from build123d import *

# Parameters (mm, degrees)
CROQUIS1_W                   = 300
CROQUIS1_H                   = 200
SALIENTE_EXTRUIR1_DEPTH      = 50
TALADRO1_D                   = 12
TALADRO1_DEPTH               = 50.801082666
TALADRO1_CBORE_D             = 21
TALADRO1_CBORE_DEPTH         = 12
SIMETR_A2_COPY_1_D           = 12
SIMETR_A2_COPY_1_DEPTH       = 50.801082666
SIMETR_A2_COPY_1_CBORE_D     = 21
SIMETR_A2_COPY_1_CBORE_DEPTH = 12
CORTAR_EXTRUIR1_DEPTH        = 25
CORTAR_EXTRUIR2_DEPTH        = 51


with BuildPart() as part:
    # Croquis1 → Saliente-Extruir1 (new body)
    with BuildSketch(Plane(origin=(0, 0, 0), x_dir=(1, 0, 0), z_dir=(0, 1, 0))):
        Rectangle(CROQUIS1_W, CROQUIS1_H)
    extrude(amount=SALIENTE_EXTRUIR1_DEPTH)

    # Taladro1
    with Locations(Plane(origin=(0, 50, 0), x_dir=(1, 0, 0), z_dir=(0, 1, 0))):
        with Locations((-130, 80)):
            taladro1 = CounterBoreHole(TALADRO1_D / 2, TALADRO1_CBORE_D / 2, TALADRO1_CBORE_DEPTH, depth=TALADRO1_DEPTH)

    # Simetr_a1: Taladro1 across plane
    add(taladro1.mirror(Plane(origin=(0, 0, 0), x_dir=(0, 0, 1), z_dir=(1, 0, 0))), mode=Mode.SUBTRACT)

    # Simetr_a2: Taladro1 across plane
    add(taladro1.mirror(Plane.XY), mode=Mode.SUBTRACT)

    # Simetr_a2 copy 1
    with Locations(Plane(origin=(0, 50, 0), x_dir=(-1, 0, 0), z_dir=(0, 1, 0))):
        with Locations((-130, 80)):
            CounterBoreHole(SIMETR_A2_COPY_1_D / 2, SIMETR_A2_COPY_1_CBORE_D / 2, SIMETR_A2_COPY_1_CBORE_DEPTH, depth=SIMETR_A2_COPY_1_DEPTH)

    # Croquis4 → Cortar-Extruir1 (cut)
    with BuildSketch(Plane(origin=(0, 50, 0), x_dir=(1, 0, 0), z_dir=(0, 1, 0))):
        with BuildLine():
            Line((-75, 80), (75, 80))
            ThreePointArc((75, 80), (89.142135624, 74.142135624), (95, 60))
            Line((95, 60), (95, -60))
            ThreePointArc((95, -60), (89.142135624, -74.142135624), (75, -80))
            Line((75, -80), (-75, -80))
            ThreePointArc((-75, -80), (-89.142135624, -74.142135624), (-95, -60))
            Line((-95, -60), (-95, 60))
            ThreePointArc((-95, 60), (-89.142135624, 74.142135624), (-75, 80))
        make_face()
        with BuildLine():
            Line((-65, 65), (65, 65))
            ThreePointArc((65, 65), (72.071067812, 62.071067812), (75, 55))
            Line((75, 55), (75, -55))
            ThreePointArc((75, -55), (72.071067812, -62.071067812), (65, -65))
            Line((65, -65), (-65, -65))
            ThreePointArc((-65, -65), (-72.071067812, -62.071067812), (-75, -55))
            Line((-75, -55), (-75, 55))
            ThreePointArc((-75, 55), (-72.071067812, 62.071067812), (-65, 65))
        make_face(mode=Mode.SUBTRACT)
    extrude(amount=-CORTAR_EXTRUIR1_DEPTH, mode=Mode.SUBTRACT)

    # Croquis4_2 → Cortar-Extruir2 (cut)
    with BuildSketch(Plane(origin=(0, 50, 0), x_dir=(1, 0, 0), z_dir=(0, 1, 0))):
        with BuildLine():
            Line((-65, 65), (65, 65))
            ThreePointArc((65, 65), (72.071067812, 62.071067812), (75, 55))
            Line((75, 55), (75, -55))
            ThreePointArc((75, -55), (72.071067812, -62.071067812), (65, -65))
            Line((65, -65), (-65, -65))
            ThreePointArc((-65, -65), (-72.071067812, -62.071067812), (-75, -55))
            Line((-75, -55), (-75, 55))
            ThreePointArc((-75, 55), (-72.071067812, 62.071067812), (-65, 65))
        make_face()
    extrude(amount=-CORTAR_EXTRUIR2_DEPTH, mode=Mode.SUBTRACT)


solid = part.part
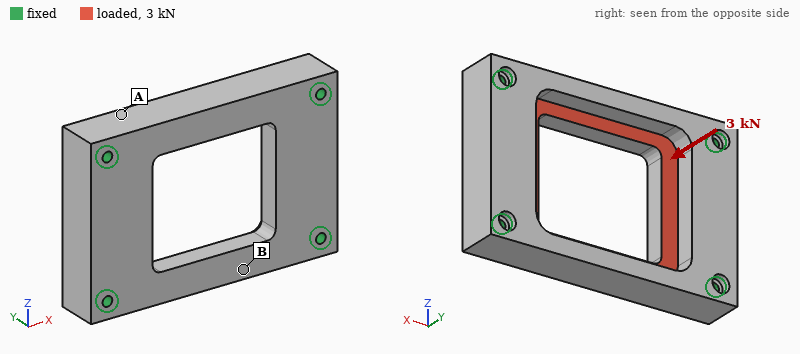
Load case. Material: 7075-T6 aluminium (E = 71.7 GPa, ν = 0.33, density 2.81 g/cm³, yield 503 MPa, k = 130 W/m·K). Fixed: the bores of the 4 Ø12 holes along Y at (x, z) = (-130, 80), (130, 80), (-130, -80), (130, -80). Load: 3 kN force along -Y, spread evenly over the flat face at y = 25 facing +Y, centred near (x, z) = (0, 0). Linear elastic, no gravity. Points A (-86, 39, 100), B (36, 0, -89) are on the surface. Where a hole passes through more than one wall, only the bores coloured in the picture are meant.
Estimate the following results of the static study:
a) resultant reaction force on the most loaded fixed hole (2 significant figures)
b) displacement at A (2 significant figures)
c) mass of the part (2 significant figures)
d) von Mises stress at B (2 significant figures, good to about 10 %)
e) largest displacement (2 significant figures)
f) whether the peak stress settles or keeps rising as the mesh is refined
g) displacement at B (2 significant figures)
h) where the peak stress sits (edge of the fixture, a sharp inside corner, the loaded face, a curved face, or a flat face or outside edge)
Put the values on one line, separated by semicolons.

750 N; 1.8 µm; 4.9 kg; 1.1 MPa; 6.1 µm; keeps rising; 4.1 µm; edge of the fixture
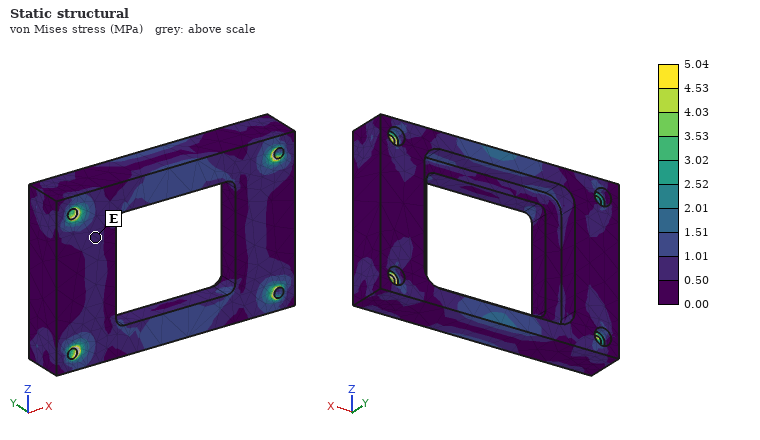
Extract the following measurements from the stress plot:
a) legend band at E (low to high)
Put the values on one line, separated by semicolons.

0.50 to 1.01 MPa
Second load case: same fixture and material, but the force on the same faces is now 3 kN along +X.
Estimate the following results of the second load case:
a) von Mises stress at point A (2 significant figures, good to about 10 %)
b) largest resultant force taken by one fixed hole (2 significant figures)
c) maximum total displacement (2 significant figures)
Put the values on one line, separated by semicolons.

0.27 MPa; 770 N; 0.79 µm
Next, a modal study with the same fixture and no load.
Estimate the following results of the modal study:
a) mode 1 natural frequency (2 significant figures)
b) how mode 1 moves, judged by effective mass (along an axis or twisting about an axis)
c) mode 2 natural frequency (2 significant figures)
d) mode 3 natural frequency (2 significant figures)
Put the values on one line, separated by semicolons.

2900 Hz; along Y; 3100 Hz; 3400 Hz
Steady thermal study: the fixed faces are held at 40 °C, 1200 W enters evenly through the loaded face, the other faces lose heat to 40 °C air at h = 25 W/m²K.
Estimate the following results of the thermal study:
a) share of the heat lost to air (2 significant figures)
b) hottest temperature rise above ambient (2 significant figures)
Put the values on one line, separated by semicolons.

10.0 %; 73 K
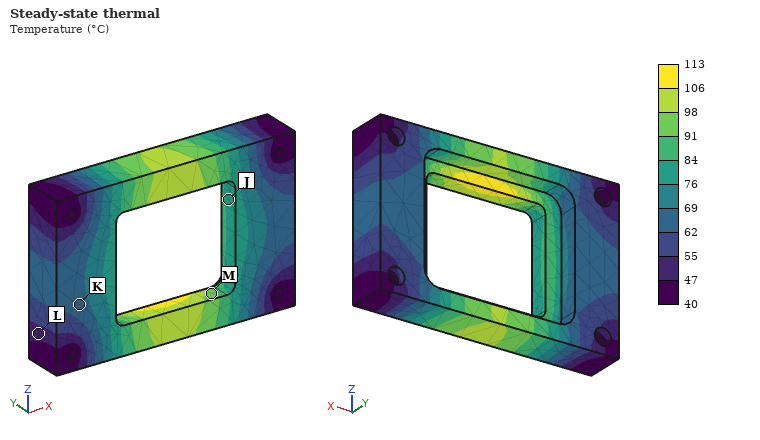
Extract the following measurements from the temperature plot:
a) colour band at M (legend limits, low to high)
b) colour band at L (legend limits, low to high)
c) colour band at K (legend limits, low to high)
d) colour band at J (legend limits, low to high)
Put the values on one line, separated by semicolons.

91 to 98 °C; 47 to 55 °C; 62 to 69 °C; 76 to 84 °C
